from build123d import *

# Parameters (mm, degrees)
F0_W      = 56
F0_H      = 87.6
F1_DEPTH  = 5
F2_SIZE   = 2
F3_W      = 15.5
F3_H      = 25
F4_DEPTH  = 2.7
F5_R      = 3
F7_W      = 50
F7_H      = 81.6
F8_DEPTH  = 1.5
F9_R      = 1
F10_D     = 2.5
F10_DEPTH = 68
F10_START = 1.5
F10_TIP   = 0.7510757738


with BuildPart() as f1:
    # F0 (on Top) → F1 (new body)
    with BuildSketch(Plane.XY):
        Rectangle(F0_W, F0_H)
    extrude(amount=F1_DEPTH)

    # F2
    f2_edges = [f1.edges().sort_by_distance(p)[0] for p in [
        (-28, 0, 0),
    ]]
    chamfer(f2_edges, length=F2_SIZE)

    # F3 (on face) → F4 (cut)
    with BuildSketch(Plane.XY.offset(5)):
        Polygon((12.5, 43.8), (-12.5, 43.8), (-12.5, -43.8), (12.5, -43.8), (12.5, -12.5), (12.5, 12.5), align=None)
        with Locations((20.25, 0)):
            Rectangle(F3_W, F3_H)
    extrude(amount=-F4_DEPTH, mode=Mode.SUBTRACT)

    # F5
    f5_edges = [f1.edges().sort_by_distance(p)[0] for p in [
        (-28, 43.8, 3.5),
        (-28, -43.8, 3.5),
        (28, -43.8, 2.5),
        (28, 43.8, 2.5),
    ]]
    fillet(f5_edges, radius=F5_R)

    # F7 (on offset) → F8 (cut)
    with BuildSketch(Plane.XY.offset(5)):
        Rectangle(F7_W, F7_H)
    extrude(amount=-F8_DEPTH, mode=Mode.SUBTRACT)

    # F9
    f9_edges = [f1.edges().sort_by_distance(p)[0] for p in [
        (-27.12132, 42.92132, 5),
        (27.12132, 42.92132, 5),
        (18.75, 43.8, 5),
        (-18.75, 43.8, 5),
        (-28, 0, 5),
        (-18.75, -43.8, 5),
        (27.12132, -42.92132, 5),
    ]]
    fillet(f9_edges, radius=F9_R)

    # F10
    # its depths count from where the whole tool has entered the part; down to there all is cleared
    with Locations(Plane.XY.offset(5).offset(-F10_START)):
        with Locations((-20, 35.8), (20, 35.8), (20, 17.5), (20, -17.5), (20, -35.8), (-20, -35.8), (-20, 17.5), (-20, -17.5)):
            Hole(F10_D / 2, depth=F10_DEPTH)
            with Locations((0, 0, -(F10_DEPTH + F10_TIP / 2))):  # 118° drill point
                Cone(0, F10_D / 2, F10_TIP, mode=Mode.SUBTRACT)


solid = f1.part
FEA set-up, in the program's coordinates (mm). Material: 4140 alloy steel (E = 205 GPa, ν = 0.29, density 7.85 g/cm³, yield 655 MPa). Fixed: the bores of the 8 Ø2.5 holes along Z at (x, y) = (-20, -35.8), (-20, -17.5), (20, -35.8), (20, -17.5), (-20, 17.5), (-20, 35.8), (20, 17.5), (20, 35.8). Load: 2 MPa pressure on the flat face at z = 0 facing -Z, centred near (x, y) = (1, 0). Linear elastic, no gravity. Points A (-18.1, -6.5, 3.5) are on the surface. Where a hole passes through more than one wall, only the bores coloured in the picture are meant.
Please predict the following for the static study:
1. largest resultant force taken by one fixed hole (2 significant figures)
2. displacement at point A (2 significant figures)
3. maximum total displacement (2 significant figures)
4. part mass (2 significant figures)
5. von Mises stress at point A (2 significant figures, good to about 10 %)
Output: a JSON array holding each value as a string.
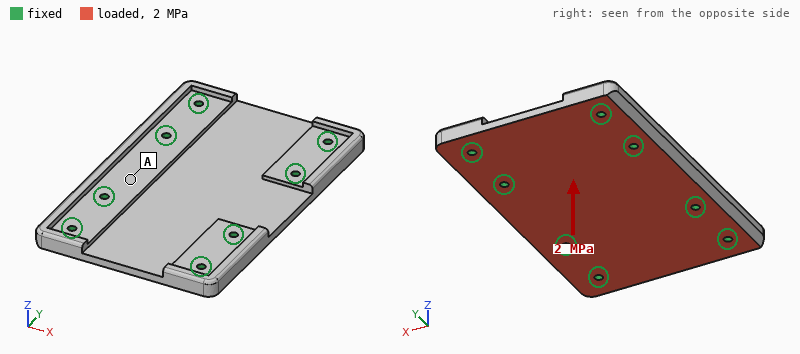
["1.8 kN", "18 µm", "67 µm", "110 g", "71 MPa"]
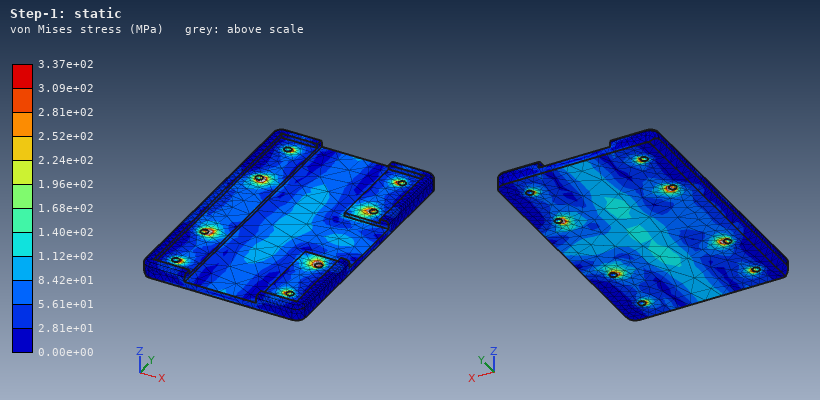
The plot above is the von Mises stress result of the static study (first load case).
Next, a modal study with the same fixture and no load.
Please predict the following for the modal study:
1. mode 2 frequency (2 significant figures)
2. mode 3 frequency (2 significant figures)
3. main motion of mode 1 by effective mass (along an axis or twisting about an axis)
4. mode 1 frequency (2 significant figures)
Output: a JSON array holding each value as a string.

["10 kHz", "11 kHz", "along Z", "8000 Hz"]
